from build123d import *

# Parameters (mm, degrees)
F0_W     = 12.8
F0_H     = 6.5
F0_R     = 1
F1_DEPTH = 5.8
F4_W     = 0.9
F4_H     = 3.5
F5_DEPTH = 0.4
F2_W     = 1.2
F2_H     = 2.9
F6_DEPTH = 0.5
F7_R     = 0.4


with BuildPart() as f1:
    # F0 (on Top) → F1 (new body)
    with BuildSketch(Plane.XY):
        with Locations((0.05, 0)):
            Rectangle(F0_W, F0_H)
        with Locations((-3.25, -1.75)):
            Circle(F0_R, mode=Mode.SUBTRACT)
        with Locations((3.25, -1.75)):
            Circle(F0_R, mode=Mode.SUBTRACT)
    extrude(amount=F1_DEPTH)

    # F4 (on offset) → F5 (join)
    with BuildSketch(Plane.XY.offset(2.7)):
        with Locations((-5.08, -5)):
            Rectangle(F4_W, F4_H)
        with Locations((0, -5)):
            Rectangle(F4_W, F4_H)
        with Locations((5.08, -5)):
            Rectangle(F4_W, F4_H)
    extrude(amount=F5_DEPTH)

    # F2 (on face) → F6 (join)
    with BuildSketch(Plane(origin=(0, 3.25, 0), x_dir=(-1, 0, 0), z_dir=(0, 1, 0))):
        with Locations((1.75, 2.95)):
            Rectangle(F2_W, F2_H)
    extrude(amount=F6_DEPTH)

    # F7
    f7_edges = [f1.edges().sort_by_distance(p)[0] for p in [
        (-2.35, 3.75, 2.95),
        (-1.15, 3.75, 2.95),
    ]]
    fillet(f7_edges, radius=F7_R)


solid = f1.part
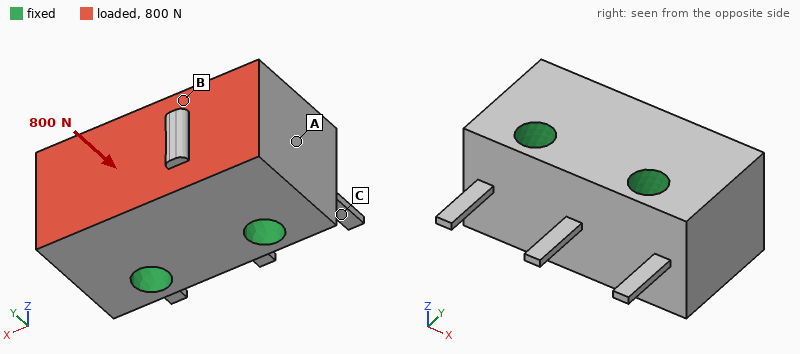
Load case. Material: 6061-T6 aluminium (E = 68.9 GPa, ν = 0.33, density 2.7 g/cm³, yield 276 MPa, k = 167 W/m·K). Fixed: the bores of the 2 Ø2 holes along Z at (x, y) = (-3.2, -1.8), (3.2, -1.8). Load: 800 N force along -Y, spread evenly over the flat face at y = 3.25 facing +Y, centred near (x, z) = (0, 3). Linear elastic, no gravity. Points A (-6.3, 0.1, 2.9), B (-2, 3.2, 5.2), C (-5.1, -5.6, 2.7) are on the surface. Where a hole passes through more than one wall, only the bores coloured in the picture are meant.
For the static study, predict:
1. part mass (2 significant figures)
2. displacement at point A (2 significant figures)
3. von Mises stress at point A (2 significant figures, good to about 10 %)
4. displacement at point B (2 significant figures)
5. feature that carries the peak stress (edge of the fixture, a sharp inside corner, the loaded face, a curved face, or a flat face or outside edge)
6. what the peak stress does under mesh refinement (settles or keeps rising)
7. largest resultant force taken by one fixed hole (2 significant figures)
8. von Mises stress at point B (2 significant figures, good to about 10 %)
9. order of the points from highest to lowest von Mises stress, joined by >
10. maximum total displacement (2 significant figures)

1.2 g
0.69 µm
5.9 MPa
0.79 µm
edge of the fixture
keeps rising
420 N
13 MPa
B > A > C
1.3 µm
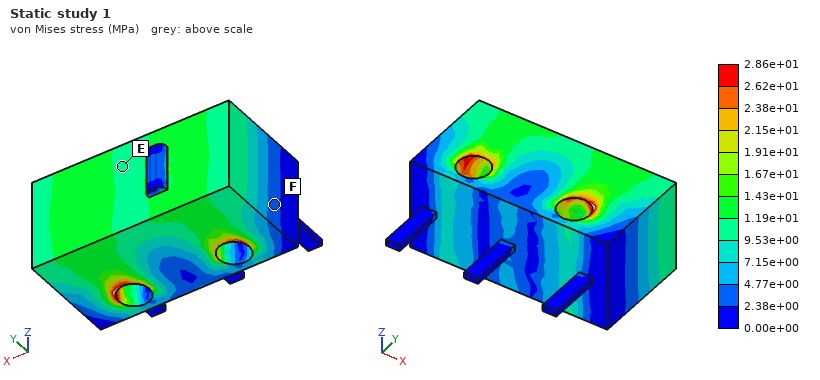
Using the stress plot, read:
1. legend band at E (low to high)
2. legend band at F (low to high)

9.53e+00 to 1.19e+01 MPa
2.38e+00 to 4.77e+00 MPa
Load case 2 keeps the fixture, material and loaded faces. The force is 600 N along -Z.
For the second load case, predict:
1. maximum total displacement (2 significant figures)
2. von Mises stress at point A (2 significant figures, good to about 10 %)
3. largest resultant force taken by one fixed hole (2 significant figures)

4.3 µm
9.3 MPa
310 N
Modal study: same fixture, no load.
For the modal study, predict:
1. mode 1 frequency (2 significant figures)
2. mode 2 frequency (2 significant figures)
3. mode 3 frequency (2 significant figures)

25 kHz
25 kHz
26 kHz
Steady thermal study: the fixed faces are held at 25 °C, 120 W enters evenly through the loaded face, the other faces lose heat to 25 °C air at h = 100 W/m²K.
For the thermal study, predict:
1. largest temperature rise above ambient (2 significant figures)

48 K
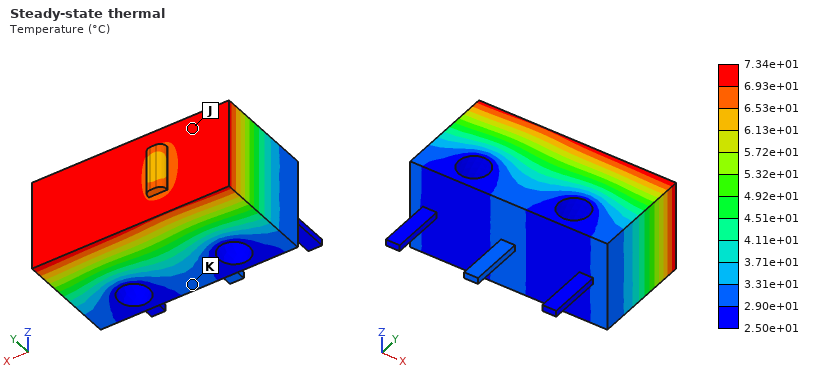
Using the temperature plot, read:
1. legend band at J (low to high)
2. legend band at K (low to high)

6.93e+01 to 7.34e+01 °C
2.90e+01 to 3.31e+01 °C
